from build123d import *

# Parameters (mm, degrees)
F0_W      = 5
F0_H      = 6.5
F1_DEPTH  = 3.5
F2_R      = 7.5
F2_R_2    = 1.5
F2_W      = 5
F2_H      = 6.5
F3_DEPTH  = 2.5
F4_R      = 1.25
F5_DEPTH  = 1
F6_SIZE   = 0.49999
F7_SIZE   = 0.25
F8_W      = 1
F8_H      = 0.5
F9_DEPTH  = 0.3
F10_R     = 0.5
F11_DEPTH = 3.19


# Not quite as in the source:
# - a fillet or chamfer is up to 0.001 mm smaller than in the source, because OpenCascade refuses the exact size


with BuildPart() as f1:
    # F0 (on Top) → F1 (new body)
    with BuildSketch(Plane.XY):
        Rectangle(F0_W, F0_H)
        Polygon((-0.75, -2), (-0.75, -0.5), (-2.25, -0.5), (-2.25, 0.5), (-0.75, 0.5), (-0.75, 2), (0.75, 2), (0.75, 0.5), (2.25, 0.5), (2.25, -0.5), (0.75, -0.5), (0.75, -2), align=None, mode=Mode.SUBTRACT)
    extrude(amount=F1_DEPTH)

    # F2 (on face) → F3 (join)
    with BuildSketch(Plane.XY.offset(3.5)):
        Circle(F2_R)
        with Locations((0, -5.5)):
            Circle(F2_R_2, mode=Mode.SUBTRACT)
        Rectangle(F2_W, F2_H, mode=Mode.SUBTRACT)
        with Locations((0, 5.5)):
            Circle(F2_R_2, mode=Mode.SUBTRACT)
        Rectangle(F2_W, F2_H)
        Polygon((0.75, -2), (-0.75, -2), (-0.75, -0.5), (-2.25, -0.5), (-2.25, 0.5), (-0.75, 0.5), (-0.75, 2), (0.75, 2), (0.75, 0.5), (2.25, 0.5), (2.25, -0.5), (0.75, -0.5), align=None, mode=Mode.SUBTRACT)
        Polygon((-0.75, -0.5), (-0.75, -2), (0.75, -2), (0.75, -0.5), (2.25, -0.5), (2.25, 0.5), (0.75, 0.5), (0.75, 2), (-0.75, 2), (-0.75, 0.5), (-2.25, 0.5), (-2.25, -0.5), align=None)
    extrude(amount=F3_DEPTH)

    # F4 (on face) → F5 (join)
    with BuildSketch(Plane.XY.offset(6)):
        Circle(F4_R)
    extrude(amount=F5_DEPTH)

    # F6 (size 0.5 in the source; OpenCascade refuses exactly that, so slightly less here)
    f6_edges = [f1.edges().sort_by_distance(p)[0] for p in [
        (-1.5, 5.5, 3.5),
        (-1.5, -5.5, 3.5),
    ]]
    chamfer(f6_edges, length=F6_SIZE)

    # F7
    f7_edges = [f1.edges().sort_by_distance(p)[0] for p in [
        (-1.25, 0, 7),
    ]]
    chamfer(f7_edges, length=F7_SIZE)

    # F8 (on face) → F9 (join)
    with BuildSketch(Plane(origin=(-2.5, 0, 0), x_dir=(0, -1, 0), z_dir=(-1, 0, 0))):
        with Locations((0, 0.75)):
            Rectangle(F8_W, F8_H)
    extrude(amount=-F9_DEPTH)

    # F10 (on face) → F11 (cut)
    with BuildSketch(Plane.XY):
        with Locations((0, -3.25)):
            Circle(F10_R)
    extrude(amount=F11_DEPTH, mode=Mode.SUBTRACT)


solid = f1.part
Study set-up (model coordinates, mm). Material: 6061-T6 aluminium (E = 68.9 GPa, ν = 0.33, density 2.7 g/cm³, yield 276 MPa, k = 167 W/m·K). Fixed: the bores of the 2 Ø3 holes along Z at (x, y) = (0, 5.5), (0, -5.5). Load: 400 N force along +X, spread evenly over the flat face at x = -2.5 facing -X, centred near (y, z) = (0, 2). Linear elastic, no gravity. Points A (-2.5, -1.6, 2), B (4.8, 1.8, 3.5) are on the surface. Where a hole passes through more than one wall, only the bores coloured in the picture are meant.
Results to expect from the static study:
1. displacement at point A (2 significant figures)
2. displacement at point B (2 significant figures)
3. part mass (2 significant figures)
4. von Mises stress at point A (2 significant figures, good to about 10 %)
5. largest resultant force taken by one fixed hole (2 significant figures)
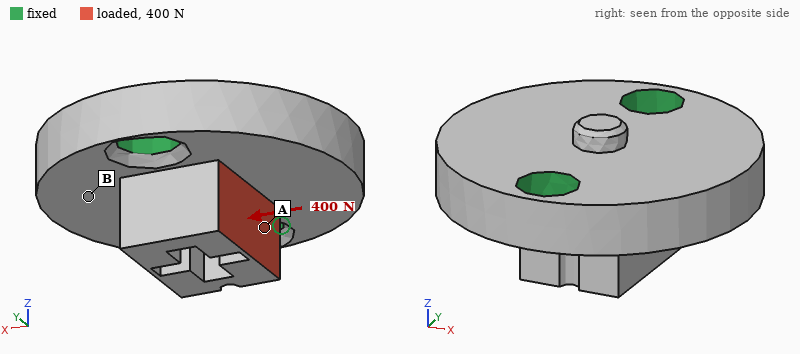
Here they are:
8.3 µm
4.8 µm
1.3 g
35 MPa
200 N
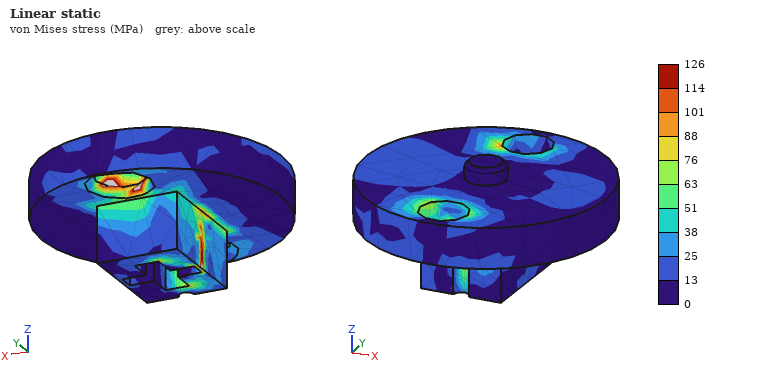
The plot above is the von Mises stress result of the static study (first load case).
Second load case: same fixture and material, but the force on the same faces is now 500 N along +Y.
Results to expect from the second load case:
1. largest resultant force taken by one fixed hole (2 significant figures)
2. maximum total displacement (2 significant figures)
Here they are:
320 N
14 µm
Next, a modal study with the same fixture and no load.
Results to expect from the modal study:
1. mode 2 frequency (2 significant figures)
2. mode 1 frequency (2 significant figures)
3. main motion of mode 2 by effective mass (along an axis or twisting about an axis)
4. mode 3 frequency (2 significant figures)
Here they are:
50 kHz
38 kHz
along Z
93 kHz
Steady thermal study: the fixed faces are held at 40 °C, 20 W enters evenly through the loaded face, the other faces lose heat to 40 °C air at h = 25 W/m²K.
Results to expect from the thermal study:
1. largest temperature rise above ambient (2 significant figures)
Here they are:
36 K
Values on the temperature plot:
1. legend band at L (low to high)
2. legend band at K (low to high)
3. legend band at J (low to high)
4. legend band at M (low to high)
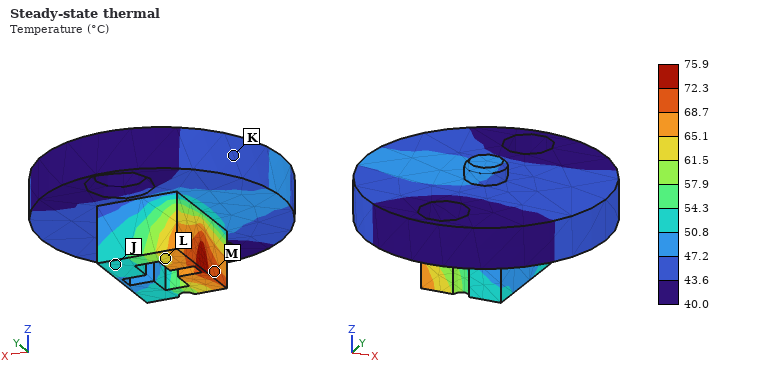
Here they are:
61.5 to 65.1 °C
43.6 to 47.2 °C
50.8 to 54.3 °C
68.7 to 72.3 °C
